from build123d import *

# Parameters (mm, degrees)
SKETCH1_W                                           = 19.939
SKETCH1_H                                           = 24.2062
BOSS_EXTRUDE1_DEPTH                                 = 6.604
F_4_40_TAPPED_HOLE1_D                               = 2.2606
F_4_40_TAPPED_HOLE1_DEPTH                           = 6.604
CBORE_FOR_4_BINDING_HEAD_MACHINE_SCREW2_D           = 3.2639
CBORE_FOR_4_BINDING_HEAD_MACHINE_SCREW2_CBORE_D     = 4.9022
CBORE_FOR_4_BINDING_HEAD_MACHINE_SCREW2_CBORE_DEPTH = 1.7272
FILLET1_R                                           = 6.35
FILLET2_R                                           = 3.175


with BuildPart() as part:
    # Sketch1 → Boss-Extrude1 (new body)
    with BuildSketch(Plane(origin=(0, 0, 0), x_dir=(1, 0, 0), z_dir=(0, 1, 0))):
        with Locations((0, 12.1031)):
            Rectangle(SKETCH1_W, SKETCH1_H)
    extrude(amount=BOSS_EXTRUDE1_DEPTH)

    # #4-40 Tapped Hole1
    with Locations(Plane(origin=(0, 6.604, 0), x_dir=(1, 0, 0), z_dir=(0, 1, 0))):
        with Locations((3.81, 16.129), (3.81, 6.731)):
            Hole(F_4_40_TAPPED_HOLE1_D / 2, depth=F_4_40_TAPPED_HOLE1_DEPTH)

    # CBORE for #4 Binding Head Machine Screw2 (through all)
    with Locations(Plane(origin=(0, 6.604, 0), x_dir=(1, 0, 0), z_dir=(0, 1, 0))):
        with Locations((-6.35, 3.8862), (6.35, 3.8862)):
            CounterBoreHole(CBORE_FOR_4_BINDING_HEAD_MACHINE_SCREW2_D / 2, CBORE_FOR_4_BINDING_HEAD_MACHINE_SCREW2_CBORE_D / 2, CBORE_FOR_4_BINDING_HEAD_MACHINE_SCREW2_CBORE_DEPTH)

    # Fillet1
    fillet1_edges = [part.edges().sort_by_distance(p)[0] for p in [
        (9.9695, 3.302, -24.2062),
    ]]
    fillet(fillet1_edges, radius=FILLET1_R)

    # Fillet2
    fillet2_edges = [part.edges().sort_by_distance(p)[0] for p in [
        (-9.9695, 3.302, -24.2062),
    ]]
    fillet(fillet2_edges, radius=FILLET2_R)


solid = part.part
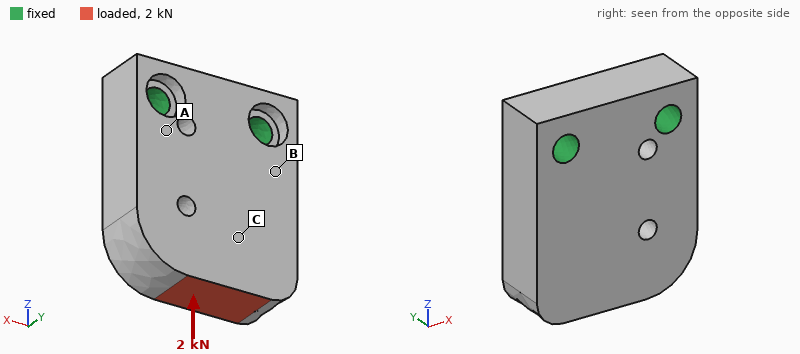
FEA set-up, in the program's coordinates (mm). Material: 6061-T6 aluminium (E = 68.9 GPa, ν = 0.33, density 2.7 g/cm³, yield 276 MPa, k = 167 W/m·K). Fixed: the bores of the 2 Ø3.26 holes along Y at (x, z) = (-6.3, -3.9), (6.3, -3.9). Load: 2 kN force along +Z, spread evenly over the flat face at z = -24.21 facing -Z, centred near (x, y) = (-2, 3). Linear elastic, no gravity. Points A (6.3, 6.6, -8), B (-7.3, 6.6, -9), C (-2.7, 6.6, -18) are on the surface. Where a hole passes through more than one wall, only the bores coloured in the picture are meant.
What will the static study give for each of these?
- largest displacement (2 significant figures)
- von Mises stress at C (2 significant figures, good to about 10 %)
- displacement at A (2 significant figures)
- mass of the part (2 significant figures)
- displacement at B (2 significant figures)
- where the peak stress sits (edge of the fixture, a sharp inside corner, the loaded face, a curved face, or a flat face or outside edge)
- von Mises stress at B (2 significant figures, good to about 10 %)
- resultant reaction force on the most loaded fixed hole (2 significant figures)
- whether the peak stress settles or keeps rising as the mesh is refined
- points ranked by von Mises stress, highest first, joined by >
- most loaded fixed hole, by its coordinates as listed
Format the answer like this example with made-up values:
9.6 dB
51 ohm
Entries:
10 µm
27 MPa
2.4 µm
7.9 g
3.5 µm
edge of the fixture
16 MPa
1.3 kN
keeps rising
C > B > A
(-6.3, -3.9)
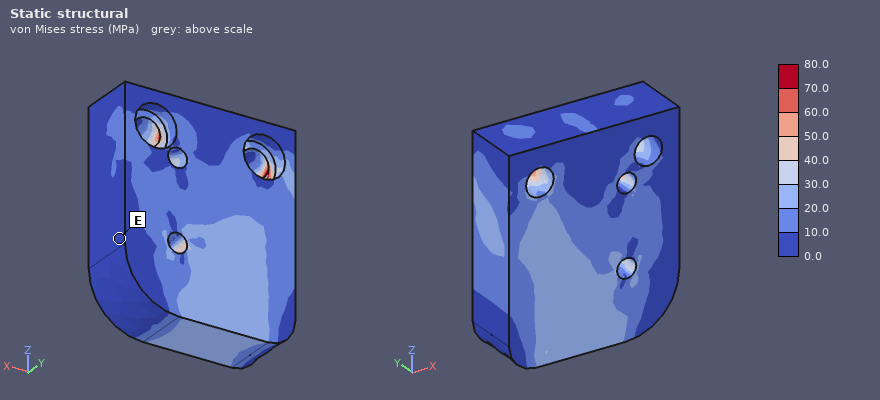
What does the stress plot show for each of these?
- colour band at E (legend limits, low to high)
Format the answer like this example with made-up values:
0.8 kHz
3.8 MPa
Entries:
0.0 to 10.0 MPa
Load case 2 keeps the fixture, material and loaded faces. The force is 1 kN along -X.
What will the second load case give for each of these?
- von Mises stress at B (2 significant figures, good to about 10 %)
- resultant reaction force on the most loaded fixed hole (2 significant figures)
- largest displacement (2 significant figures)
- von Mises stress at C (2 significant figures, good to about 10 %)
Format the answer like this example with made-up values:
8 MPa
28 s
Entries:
16 MPa
1.5 kN
20 µm
17 MPa
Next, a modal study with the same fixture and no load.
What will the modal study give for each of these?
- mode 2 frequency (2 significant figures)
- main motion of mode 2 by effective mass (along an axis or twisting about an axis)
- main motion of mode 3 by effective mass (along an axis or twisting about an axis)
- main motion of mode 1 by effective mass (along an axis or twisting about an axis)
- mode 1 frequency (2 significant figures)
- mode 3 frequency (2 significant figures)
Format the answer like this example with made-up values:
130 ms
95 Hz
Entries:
24 kHz
along X
along X
along Y
10 kHz
26 kHz
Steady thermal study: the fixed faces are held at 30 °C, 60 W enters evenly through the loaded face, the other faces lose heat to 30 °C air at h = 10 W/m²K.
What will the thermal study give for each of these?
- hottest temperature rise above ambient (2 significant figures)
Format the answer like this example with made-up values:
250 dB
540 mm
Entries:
69 K
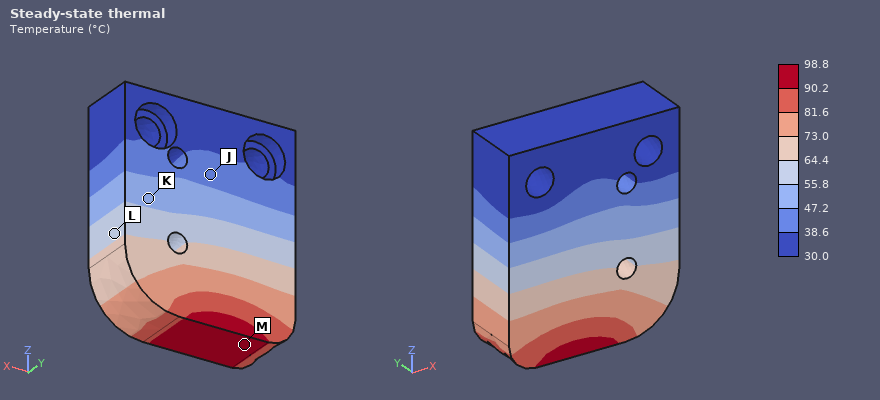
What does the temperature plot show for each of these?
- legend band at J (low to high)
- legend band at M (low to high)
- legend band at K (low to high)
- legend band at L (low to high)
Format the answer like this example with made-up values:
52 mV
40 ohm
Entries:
38.6 to 47.2 °C
90.2 to 98.8 °C
47.2 to 55.8 °C
55.8 to 64.4 °C
